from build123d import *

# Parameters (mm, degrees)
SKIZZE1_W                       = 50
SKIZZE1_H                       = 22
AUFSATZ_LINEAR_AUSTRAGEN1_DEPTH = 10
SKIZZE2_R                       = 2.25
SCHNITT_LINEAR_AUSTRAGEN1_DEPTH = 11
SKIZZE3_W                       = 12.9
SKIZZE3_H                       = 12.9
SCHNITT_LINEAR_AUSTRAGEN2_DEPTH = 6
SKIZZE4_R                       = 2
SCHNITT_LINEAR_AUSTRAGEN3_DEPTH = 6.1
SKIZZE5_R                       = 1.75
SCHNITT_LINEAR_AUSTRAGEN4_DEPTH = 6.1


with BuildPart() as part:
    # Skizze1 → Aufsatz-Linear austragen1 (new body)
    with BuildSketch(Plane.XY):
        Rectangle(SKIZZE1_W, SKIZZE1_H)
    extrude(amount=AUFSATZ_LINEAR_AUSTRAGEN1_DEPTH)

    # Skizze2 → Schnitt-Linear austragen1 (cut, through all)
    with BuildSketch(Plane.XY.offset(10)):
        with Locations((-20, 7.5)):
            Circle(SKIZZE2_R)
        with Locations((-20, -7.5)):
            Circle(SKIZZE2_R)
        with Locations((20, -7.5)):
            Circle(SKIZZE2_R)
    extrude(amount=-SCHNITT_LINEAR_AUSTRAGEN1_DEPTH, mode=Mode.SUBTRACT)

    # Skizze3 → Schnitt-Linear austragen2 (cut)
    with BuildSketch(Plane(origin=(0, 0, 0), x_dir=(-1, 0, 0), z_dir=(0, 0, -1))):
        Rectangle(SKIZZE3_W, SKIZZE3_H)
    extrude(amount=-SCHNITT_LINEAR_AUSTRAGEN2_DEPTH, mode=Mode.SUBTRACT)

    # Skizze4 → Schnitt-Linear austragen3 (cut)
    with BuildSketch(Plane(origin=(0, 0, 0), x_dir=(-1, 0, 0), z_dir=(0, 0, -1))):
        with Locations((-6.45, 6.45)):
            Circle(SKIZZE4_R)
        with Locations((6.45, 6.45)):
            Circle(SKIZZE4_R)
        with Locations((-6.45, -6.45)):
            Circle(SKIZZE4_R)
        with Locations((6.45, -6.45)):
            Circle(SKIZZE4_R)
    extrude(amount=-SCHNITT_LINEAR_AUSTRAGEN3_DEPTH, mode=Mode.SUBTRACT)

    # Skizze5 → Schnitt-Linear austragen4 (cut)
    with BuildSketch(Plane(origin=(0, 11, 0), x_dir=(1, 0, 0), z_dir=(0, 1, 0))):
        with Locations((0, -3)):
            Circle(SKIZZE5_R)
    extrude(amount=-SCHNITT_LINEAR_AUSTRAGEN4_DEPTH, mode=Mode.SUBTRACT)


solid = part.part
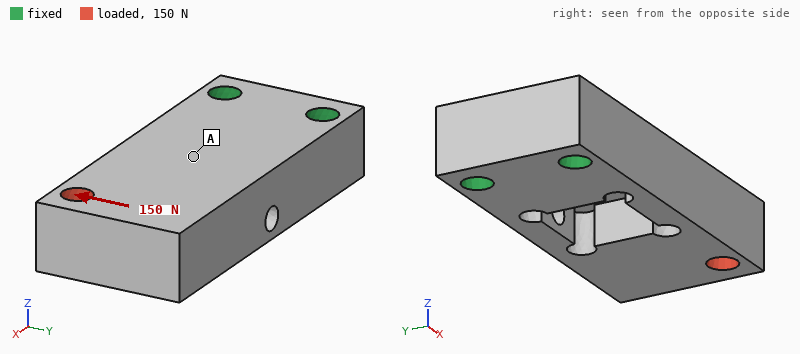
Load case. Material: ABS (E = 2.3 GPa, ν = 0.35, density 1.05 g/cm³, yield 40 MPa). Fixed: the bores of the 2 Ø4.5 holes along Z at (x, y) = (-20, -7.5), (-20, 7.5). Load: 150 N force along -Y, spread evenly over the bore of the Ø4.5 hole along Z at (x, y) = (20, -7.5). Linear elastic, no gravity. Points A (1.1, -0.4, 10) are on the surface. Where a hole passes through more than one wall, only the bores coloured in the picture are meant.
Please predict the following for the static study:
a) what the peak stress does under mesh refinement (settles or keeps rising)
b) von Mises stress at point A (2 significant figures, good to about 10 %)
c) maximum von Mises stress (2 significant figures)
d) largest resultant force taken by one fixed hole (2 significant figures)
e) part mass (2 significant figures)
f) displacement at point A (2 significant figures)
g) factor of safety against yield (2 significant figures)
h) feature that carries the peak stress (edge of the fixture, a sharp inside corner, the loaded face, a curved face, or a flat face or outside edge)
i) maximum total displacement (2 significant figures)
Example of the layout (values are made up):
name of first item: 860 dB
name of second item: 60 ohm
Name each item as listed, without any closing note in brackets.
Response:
what the peak stress does under mesh refinement: settles
von Mises stress at point A: 1.5 MPa
maximum von Mises stress: 18 MPa
largest resultant force taken by one fixed hole: 360 N
part mass: 9.7 g
displacement at point A: 0.076 mm
factor of safety against yield: 2.2
feature that carries the peak stress: a curved face
maximum total displacement: 0.36 mm
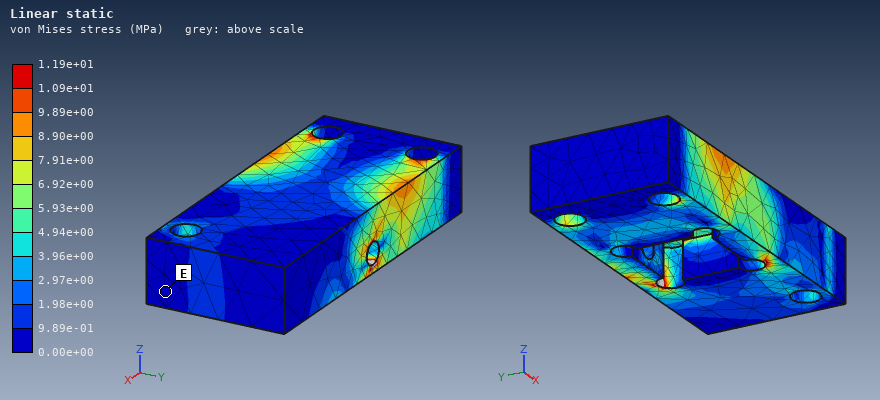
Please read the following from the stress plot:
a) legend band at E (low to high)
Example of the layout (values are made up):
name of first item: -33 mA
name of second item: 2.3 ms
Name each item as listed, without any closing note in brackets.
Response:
legend band at E: 0.00e+00 to 9.89e-01 MPa
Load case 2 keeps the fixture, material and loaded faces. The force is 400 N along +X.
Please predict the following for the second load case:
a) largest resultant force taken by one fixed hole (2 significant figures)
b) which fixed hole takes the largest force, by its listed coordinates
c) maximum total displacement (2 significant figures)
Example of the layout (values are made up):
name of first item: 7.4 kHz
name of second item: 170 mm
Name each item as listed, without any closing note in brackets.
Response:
largest resultant force taken by one fixed hole: 390 N
which fixed hole takes the largest force, by its listed coordinates: (-20, -7.5)
maximum total displacement: 0.30 mm
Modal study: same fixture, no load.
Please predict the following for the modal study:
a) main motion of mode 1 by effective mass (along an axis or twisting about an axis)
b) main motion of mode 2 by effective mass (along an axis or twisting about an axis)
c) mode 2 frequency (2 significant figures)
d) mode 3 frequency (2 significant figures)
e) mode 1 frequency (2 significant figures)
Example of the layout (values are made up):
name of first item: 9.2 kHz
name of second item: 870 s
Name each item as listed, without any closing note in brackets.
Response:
main motion of mode 1 by effective mass: along Z
main motion of mode 2 by effective mass: along Y
mode 2 frequency: 1900 Hz
mode 3 frequency: 3000 Hz
mode 1 frequency: 990 Hz
